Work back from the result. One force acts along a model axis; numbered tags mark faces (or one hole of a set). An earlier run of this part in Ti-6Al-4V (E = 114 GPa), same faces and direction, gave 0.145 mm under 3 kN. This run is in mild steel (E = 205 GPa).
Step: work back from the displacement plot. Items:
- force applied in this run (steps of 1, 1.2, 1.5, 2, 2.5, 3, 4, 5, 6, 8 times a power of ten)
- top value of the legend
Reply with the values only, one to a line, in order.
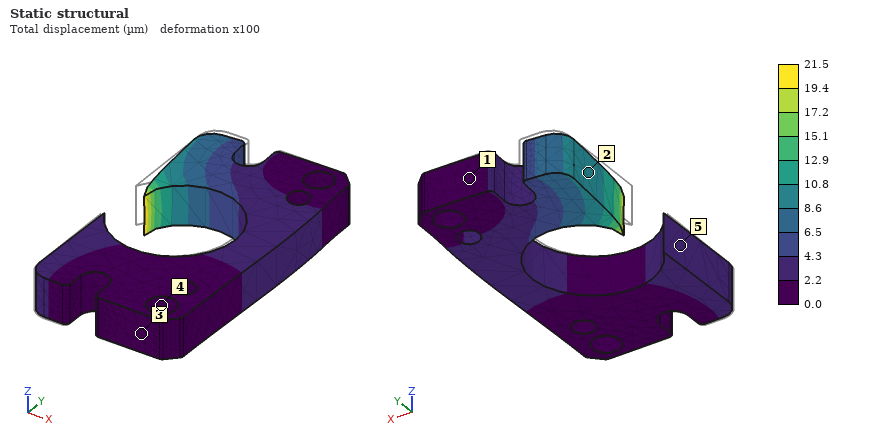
800 N
21.5 µm
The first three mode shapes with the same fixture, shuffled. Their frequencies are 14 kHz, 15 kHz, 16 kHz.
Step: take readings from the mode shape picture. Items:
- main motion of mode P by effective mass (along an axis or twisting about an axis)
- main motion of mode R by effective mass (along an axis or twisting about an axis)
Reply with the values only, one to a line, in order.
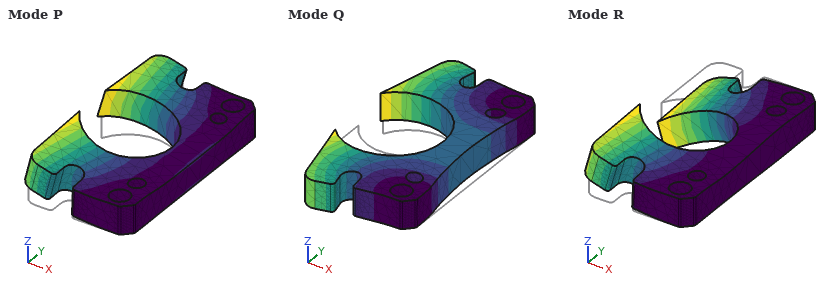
along Z
twisting about X
